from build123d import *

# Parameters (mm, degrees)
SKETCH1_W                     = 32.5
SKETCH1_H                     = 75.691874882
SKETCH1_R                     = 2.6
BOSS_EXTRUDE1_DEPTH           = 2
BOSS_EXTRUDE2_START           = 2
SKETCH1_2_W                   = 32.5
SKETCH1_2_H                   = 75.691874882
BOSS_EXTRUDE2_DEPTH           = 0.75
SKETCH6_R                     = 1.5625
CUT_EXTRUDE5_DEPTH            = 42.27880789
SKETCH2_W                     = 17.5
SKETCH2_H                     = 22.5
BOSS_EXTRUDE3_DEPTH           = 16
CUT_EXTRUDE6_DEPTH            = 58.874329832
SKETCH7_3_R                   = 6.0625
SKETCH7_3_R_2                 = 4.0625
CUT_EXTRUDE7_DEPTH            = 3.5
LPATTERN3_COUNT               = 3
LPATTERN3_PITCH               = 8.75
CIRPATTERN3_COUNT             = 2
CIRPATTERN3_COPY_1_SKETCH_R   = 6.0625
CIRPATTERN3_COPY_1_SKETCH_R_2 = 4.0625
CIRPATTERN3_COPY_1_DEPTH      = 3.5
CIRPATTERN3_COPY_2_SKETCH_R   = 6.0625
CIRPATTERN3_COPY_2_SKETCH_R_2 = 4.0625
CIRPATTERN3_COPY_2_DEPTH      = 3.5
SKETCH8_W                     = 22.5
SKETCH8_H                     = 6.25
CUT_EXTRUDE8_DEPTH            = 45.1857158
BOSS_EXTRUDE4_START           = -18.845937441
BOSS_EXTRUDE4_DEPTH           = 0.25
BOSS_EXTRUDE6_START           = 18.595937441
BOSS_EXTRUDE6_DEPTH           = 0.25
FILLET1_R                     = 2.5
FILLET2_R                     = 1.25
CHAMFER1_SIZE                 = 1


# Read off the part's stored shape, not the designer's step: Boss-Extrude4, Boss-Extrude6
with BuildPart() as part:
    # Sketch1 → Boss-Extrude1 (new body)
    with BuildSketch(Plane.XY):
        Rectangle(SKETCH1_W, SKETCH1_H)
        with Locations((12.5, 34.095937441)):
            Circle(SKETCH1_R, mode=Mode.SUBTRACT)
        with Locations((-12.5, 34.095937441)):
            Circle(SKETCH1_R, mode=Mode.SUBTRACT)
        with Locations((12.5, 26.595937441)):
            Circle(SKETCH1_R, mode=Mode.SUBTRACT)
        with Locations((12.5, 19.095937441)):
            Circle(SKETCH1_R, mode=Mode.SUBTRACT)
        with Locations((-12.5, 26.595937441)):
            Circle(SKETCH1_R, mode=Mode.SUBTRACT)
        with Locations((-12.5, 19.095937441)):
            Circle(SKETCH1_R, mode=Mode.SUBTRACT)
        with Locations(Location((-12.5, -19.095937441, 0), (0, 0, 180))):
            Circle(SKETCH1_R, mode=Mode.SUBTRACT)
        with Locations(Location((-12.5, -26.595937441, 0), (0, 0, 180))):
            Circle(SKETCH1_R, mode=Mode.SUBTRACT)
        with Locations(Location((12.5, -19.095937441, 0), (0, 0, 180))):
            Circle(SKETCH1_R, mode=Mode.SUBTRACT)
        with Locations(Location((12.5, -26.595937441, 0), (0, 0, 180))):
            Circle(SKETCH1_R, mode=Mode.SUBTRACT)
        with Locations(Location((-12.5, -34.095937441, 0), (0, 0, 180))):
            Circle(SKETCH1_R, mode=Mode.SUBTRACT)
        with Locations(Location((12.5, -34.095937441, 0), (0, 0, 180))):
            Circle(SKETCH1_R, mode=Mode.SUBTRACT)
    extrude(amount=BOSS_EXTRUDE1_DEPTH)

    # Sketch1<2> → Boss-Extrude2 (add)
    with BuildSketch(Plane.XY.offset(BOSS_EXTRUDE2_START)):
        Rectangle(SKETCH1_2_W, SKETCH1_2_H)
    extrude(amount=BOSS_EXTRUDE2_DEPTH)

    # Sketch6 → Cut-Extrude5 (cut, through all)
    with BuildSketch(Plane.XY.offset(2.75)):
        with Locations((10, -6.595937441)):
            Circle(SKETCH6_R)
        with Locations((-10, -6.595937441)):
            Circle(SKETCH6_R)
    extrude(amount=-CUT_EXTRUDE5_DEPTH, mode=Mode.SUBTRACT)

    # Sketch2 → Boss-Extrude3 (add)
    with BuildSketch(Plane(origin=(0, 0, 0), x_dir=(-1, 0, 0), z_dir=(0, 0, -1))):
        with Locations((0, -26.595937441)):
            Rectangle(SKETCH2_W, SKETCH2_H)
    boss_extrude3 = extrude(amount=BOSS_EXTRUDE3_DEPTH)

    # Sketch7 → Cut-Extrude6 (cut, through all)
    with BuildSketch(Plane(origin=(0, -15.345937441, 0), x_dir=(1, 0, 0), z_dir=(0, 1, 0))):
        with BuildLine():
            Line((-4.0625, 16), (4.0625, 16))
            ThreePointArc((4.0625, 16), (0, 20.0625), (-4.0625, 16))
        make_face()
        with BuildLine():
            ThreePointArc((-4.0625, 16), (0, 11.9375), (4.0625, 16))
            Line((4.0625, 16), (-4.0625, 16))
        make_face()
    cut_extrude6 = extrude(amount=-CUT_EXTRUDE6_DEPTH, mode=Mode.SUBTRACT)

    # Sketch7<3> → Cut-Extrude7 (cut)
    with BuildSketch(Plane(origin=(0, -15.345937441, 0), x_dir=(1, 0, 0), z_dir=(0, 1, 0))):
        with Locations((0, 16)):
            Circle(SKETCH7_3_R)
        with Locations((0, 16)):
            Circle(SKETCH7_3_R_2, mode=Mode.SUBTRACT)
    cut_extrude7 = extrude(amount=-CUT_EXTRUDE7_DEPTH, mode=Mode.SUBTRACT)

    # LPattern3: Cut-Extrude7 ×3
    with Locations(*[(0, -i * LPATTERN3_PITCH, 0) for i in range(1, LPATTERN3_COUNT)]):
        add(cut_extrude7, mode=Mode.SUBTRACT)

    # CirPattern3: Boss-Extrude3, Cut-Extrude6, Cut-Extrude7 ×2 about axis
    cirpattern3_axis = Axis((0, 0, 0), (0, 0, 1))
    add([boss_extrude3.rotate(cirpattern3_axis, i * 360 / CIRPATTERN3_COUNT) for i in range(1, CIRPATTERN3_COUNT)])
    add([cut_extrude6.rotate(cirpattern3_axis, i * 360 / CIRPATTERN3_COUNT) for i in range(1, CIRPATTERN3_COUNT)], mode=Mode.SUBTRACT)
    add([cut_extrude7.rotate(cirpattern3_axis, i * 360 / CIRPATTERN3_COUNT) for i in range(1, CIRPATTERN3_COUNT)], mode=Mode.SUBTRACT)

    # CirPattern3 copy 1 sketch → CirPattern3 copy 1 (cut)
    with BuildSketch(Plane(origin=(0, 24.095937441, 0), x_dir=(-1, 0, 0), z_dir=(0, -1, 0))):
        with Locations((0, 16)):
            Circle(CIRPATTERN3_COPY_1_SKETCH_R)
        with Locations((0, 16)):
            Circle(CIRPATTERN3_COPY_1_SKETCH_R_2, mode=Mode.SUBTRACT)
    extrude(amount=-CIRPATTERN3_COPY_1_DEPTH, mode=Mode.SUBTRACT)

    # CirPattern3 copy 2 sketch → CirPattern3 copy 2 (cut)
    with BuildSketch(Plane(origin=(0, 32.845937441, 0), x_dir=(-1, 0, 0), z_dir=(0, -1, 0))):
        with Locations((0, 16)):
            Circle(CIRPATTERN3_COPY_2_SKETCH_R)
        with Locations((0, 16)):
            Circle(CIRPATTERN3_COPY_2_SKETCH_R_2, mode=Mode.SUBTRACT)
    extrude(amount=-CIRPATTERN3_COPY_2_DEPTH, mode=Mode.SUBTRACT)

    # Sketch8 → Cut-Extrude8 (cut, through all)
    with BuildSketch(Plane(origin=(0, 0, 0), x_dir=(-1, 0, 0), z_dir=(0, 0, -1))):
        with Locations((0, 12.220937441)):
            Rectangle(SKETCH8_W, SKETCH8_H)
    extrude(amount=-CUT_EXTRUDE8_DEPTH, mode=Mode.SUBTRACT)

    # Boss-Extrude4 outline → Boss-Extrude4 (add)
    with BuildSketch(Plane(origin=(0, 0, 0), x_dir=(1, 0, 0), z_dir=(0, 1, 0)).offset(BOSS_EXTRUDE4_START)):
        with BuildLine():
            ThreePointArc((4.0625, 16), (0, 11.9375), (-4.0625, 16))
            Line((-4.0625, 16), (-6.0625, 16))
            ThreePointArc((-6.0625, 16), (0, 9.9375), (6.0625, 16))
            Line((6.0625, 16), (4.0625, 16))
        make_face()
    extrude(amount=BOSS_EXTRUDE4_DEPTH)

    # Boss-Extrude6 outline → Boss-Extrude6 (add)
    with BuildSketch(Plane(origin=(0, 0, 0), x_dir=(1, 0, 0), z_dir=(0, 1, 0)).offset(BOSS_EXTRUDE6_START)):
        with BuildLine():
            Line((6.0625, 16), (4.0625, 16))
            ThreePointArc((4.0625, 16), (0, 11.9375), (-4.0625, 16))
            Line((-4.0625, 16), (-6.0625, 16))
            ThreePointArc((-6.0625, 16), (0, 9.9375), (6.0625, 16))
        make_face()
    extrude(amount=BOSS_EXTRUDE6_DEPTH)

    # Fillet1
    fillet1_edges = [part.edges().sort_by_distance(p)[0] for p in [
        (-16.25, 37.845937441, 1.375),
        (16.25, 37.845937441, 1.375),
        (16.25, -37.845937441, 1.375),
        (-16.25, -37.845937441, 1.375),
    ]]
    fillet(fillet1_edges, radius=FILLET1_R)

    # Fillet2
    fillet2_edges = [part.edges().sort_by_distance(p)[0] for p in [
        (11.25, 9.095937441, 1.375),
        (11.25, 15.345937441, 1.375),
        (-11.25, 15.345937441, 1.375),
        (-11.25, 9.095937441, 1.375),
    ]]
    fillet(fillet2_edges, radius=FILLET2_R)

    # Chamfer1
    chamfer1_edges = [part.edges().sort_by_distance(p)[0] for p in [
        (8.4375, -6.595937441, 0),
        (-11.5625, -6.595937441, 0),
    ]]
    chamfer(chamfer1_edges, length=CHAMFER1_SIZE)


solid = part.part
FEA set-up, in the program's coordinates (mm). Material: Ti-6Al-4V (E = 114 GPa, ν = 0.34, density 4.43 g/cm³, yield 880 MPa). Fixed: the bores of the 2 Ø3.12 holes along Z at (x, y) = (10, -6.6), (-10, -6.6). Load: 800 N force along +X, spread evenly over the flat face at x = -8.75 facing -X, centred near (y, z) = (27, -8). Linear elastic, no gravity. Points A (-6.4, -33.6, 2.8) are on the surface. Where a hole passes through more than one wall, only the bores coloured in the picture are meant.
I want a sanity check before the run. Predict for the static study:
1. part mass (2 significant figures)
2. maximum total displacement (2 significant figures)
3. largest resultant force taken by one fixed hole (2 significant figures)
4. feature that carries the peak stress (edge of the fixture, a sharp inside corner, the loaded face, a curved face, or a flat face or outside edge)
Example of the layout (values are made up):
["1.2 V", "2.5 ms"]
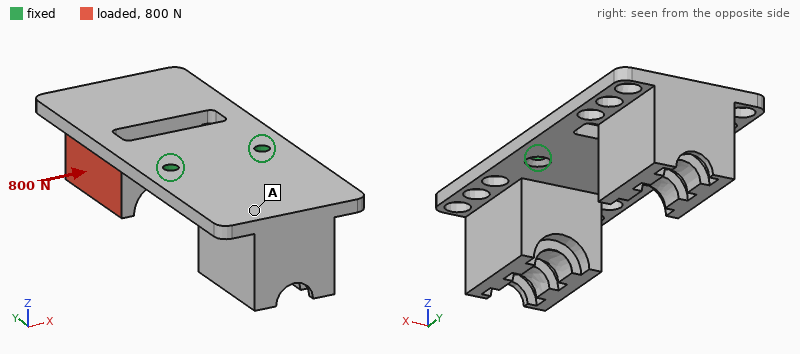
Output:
["73 g", "0.39 mm", "1.4 kN", "a curved face"]
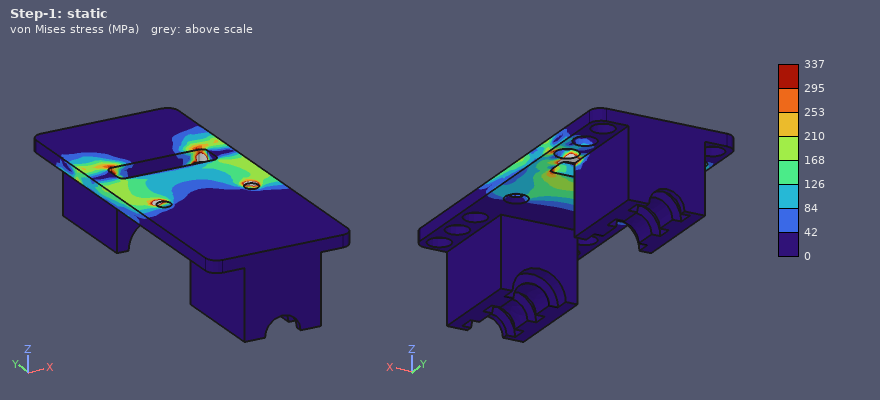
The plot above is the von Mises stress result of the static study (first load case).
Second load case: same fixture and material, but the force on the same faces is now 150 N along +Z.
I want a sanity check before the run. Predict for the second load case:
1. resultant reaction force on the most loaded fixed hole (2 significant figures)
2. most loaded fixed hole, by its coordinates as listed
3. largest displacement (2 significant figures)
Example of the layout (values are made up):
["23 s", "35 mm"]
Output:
["140 N", "(-10, -6.6)", "0.90 mm"]
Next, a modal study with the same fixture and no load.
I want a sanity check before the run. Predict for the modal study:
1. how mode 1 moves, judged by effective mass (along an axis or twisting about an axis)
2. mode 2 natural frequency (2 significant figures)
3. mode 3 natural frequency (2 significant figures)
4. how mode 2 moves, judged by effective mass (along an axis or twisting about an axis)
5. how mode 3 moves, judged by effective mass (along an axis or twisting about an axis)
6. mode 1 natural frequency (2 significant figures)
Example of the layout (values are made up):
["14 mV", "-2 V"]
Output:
["along Z", "1100 Hz", "1700 Hz", "along Z", "along X", "440 Hz"]
